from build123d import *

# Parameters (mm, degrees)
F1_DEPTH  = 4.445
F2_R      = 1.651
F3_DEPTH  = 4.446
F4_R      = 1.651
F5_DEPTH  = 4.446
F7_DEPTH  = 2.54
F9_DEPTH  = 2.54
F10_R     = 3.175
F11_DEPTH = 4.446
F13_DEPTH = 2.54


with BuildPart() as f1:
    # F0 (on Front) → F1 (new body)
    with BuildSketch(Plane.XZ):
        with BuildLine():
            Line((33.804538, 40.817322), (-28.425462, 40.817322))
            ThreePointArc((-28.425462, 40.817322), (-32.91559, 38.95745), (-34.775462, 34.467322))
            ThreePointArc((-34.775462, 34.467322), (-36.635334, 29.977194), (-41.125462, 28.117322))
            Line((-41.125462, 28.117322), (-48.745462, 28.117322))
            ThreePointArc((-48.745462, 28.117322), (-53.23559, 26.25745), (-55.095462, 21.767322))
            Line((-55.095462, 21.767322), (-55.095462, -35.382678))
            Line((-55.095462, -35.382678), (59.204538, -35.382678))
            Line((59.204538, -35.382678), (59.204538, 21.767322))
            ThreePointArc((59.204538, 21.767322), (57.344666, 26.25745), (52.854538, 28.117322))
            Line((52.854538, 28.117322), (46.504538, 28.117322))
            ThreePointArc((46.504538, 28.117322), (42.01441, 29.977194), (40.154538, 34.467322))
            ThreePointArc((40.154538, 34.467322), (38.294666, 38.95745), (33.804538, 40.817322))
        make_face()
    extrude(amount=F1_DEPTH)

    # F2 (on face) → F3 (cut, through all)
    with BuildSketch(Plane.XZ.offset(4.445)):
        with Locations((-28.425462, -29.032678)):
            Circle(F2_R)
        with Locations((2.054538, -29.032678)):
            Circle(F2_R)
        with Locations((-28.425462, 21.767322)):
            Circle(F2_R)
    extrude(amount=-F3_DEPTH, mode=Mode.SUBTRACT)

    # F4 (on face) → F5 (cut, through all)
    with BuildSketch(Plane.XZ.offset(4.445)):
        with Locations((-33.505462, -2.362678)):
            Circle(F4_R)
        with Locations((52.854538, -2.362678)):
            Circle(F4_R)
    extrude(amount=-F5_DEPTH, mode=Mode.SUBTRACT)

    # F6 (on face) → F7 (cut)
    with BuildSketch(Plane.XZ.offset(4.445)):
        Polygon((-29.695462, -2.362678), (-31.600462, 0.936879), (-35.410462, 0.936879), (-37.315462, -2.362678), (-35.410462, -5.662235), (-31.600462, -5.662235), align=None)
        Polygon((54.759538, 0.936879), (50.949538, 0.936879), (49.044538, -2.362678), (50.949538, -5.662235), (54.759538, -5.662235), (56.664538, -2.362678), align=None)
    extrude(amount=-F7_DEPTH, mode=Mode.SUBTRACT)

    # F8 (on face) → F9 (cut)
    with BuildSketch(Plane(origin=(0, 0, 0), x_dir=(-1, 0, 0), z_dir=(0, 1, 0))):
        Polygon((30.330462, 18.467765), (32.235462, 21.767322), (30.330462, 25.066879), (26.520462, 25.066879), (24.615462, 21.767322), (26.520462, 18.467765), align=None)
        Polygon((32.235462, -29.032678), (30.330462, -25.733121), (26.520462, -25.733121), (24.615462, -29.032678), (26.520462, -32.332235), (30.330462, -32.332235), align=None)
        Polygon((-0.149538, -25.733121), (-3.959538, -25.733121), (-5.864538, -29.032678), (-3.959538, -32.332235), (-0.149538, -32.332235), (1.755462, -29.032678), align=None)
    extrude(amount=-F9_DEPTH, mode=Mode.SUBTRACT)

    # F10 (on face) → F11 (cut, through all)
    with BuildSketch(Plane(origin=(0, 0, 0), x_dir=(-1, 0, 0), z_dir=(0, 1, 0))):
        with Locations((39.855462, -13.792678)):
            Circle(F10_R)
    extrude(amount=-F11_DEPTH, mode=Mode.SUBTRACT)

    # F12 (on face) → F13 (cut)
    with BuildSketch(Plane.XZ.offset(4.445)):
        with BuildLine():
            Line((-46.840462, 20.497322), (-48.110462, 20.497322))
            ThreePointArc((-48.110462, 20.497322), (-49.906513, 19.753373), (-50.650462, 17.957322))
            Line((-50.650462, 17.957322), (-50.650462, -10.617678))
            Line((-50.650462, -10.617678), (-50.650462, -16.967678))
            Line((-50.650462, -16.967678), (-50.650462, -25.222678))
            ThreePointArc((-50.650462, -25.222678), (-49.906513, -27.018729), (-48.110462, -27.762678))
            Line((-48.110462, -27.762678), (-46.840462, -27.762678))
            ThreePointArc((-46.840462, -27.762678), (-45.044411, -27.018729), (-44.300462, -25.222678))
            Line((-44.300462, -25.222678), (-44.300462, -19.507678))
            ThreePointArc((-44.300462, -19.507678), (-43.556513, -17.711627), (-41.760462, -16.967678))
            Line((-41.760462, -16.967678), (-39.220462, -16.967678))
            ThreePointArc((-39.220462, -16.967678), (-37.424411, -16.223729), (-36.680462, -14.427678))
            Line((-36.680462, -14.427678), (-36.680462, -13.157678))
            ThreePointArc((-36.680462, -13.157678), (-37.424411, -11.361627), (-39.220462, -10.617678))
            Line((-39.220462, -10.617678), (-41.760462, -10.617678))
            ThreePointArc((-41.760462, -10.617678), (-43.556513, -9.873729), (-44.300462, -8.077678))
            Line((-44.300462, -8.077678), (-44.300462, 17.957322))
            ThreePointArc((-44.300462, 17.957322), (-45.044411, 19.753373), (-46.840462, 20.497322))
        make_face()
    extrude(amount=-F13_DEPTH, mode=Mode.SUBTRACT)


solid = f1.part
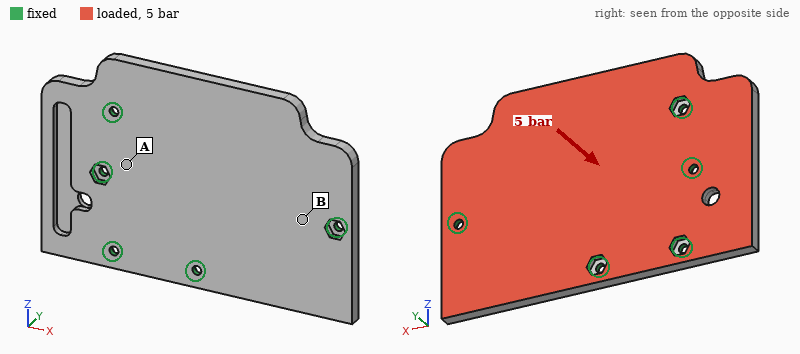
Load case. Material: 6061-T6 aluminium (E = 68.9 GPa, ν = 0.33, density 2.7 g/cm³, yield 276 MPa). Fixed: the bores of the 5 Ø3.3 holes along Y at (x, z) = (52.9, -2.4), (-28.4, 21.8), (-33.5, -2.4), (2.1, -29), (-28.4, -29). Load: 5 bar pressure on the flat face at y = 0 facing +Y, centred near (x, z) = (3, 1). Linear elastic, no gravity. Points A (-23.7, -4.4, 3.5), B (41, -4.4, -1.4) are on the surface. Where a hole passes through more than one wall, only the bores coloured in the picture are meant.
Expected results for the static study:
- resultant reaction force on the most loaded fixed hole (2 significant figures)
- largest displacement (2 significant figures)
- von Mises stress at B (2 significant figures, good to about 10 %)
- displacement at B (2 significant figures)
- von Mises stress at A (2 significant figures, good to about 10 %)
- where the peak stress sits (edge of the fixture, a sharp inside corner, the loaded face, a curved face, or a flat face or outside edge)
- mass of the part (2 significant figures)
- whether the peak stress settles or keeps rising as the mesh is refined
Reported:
1.5 kN
0.60 mm
85 MPa
0.098 mm
31 MPa
edge of the fixture
94 g
keeps rising
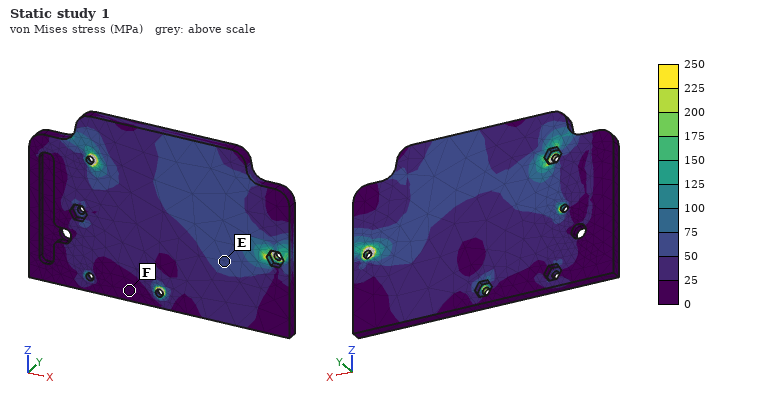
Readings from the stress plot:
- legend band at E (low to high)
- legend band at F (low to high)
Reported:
50 to 75 MPa
0 to 25 MPa
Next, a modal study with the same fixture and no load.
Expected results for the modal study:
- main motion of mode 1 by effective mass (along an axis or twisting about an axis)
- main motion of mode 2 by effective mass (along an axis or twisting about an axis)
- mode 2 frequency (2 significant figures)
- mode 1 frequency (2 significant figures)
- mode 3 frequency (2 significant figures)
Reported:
along Y
along Y
3200 Hz
1600 Hz
4300 Hz
